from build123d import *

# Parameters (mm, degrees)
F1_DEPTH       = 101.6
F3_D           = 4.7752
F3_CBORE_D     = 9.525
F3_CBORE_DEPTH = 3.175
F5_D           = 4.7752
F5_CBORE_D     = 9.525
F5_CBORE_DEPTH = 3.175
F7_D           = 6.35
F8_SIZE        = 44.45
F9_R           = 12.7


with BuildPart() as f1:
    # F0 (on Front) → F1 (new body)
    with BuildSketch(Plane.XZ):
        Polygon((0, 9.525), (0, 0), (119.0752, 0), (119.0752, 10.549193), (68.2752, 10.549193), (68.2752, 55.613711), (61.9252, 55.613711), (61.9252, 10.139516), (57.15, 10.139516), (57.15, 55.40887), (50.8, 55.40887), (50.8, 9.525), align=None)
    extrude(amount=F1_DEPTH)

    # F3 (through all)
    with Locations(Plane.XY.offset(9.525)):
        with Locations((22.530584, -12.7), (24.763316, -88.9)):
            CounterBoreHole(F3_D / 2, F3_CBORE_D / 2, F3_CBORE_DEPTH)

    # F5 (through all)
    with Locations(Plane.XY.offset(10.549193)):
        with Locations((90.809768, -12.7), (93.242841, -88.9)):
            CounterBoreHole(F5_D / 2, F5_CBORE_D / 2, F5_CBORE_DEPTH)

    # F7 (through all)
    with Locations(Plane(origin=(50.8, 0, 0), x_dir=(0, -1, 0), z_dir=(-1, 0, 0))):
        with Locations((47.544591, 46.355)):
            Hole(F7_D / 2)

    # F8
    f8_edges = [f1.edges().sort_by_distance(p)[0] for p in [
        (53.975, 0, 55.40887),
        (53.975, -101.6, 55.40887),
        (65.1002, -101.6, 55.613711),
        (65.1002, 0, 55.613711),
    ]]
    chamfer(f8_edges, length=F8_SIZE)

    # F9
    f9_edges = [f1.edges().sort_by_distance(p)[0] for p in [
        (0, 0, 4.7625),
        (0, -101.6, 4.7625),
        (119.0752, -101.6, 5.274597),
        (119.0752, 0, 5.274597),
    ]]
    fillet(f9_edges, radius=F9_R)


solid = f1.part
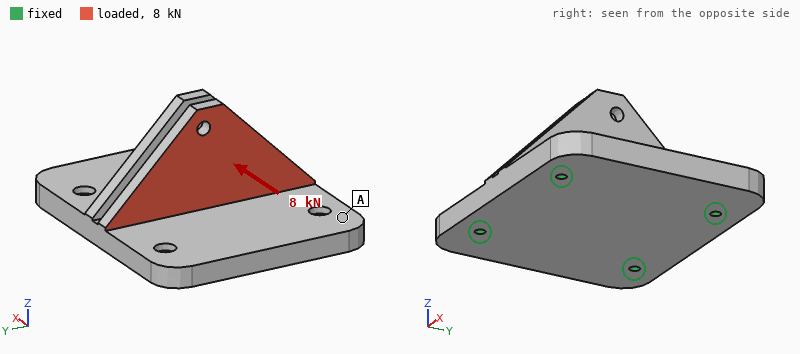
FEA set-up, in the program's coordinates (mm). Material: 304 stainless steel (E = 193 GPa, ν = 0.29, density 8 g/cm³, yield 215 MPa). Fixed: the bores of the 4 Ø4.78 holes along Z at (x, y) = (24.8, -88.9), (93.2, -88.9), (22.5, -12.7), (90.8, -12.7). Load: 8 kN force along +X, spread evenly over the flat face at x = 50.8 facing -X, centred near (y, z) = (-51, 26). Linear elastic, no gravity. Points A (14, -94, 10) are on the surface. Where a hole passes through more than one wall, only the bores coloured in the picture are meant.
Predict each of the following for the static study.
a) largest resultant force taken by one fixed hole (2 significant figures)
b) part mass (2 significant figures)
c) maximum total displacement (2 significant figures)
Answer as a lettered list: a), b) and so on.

a) 2.8 kN
b) 1.2 kg
c) 0.26 mm
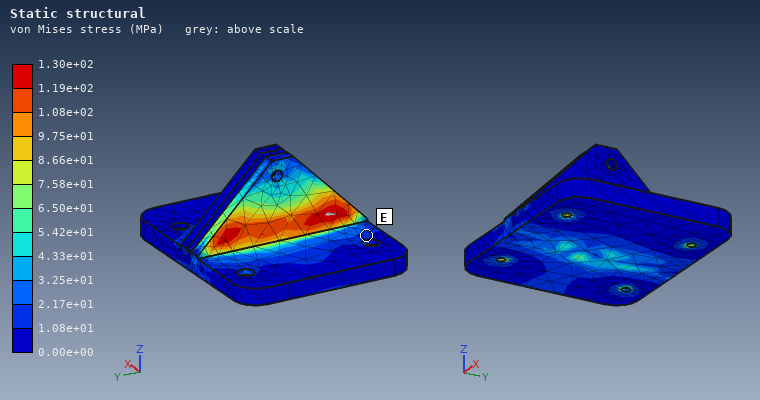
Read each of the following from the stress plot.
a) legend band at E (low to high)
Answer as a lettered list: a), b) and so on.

a) 1.08e+01 to 2.17e+01 MPa
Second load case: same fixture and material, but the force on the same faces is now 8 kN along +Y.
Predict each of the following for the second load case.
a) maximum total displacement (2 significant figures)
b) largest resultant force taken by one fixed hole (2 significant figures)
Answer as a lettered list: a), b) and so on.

a) 23 µm
b) 2.8 kN
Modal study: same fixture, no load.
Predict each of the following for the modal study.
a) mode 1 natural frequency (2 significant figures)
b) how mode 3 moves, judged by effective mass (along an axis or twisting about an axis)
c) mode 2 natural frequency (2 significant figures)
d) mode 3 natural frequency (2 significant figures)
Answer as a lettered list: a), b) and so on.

a) 3200 Hz
b) along Z
c) 3300 Hz
d) 4400 Hz
